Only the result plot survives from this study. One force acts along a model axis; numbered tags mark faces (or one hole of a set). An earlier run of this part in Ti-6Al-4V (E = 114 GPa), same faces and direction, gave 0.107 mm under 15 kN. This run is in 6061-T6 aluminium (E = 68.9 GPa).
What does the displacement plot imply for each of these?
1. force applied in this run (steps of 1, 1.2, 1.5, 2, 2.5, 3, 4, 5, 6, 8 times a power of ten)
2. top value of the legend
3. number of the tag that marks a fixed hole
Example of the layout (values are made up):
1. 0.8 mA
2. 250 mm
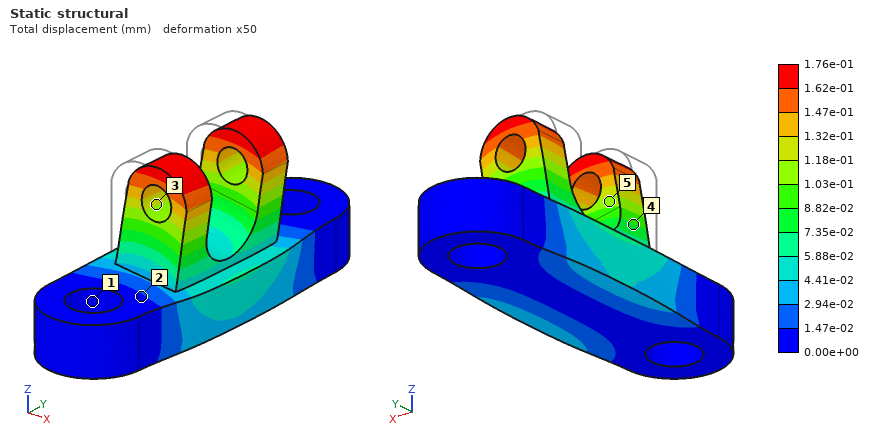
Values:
1. 15 kN
2. 1.76e-01 mm
3. 1
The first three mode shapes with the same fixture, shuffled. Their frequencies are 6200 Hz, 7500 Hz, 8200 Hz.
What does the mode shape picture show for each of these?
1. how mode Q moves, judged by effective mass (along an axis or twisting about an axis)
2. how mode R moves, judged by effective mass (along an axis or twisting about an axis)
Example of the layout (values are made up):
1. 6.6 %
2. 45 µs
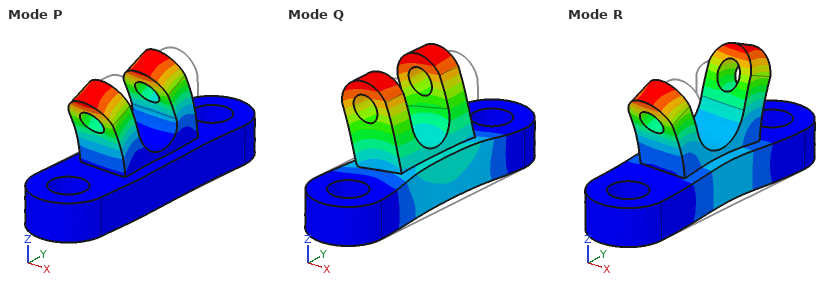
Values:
1. along X
2. along Z
